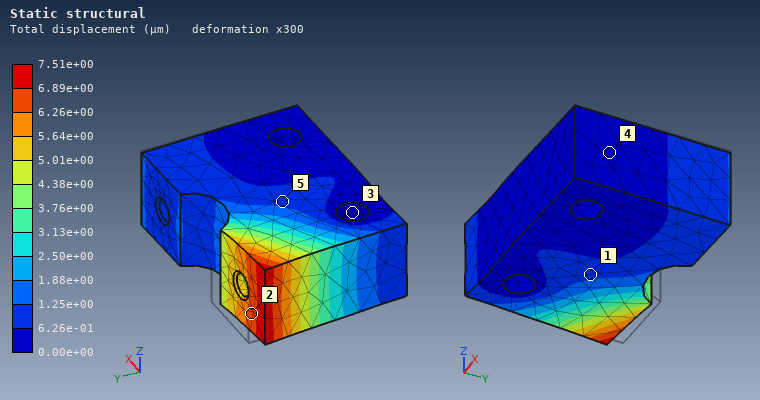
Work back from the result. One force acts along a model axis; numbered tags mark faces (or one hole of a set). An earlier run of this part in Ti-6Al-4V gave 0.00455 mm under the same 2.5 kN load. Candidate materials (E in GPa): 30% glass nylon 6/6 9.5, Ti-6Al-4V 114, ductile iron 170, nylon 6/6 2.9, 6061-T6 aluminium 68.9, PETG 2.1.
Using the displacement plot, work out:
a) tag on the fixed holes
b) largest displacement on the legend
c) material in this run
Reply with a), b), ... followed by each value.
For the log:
a) 3
b) 7.51e+00 µm
c) 6061-T6 aluminium
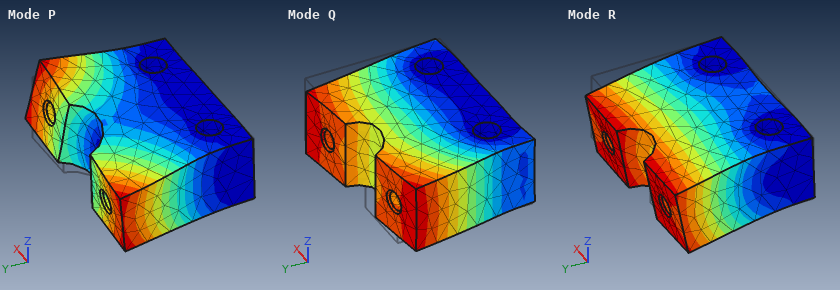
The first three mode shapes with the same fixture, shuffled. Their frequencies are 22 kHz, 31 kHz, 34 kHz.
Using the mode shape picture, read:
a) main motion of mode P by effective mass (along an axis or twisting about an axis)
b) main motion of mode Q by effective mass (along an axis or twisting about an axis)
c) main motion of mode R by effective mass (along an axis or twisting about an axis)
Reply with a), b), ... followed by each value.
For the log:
a) twisting about Y
b) along X
c) along Z
